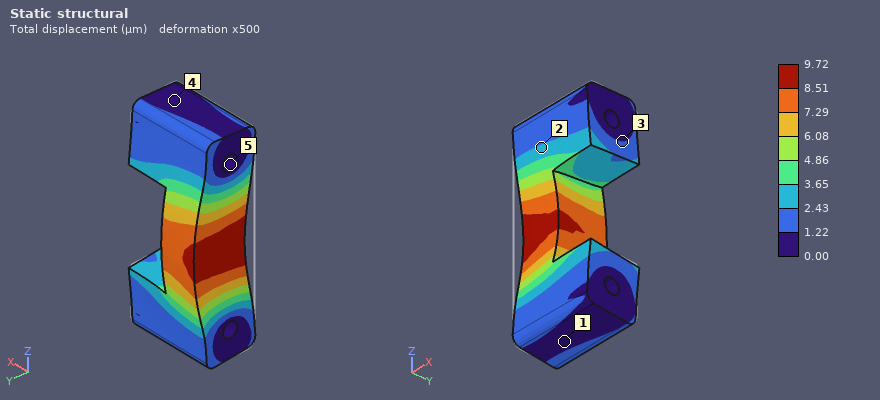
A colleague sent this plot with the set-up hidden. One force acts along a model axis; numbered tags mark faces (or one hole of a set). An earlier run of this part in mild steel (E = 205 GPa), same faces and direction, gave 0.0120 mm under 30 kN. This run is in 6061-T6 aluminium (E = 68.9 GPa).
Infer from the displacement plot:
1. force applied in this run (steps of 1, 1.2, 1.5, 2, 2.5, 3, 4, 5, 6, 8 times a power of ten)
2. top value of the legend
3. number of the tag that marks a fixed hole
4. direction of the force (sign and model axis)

8 kN
9.72 µm
5
+Y
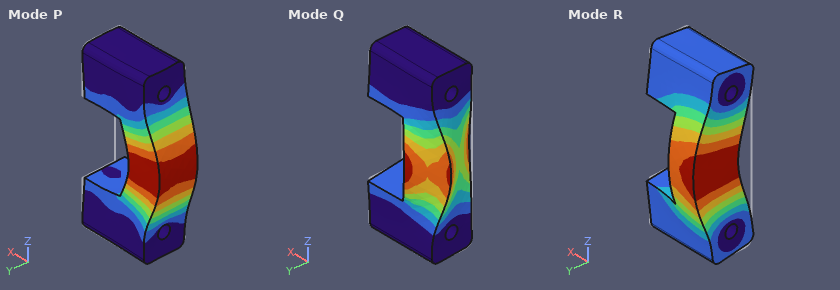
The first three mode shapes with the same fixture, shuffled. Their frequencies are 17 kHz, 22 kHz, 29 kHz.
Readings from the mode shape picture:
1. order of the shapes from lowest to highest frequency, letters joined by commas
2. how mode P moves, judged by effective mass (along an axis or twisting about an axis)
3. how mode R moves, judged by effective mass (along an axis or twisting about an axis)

R, P, Q
along X
along Y
